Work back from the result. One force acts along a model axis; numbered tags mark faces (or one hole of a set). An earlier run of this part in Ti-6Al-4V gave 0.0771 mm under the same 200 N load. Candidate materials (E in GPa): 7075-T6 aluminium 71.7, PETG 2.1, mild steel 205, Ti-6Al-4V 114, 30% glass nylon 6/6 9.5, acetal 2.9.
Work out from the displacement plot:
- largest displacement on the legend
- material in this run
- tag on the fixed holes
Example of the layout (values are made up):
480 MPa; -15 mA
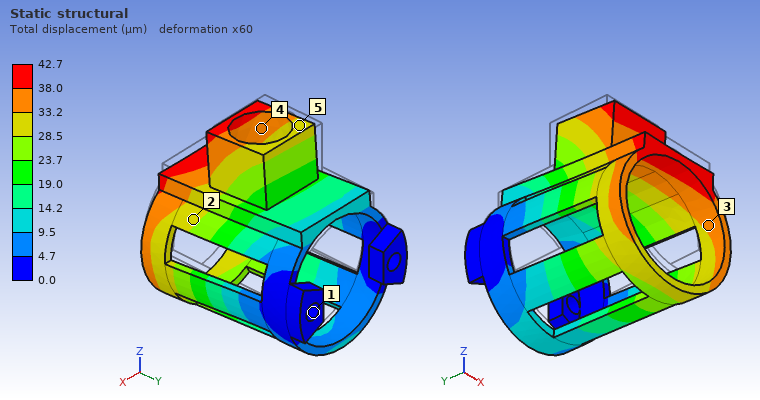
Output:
42.7 µm; mild steel; 1
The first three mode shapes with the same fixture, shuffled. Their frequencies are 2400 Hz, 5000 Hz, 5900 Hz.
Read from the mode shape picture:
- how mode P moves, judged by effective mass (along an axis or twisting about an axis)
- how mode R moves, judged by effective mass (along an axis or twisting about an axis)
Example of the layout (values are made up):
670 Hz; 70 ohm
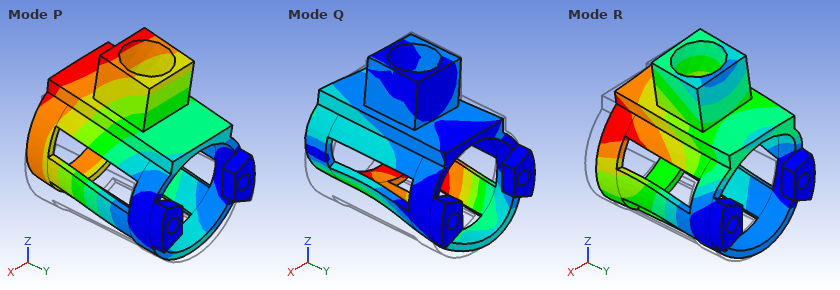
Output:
along Z; along X
